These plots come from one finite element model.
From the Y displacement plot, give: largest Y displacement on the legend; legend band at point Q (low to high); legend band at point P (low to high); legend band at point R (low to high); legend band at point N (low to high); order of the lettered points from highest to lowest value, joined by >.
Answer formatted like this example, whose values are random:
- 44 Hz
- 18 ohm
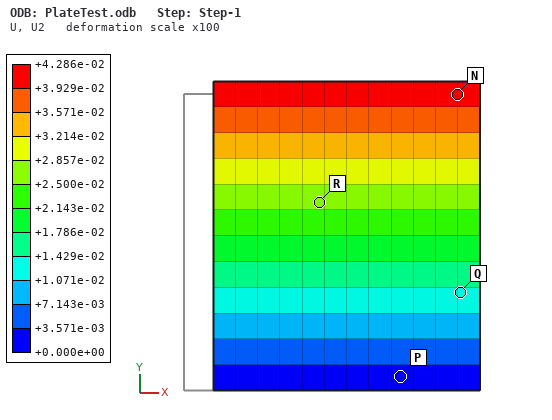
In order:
- +4.286e-02
- +1.071e-02 to +1.429e-02
- +0.000e+00 to +3.571e-03
- +2.500e-02 to +2.857e-02
- +3.929e-02 to +4.286e-02
- N > R > Q > P
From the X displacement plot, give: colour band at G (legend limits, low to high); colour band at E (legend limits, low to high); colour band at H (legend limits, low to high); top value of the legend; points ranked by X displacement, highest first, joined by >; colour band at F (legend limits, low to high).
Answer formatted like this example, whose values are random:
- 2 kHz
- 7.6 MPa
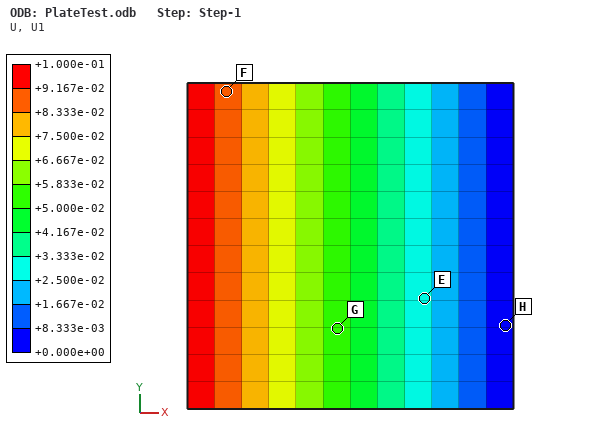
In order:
- +5.000e-02 to +5.833e-02
- +2.500e-02 to +3.333e-02
- +0.000e+00 to +8.333e-03
- +1.000e-01
- F > G > E > H
- +8.333e-02 to +9.167e-02
